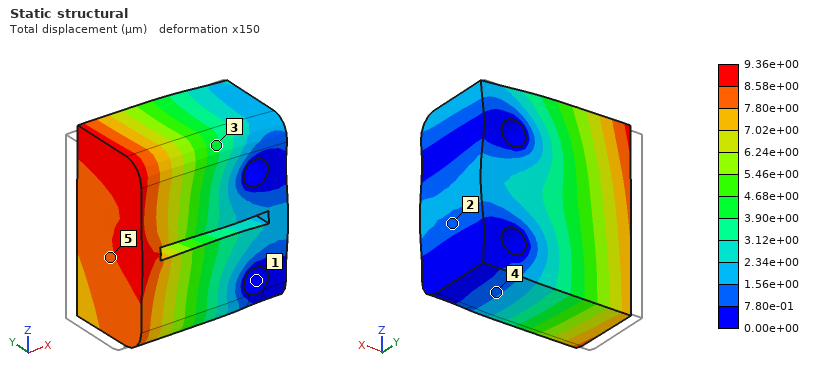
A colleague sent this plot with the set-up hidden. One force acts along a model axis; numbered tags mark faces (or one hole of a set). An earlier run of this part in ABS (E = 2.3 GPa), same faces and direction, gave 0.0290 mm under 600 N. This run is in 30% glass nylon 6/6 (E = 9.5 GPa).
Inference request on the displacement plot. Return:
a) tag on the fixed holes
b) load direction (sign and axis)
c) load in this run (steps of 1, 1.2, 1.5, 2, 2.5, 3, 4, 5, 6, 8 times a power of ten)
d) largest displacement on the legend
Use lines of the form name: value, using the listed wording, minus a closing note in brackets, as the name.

tag on the fixed holes: 1
load direction: +X
load in this run: 800 N
largest displacement on the legend: 9.36e+00 µm
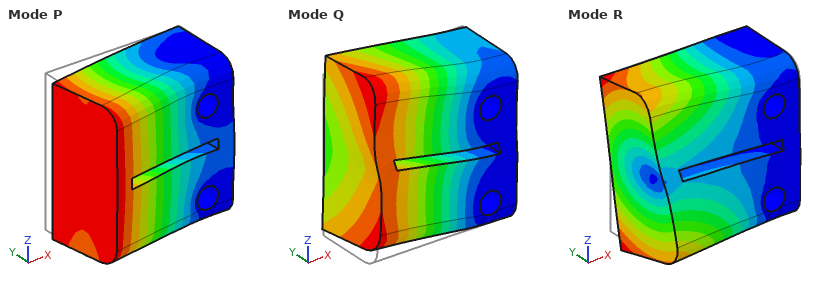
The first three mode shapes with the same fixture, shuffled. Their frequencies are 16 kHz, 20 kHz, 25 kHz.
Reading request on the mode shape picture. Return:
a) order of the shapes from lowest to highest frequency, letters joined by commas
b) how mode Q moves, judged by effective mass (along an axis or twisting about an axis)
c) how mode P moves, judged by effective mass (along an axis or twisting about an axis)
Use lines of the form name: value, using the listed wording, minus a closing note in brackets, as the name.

order of the shapes from lowest to highest frequency, letters joined by commas: P, Q, R
how mode Q moves, judged by effective mass: along Z
how mode P moves, judged by effective mass: along Y
